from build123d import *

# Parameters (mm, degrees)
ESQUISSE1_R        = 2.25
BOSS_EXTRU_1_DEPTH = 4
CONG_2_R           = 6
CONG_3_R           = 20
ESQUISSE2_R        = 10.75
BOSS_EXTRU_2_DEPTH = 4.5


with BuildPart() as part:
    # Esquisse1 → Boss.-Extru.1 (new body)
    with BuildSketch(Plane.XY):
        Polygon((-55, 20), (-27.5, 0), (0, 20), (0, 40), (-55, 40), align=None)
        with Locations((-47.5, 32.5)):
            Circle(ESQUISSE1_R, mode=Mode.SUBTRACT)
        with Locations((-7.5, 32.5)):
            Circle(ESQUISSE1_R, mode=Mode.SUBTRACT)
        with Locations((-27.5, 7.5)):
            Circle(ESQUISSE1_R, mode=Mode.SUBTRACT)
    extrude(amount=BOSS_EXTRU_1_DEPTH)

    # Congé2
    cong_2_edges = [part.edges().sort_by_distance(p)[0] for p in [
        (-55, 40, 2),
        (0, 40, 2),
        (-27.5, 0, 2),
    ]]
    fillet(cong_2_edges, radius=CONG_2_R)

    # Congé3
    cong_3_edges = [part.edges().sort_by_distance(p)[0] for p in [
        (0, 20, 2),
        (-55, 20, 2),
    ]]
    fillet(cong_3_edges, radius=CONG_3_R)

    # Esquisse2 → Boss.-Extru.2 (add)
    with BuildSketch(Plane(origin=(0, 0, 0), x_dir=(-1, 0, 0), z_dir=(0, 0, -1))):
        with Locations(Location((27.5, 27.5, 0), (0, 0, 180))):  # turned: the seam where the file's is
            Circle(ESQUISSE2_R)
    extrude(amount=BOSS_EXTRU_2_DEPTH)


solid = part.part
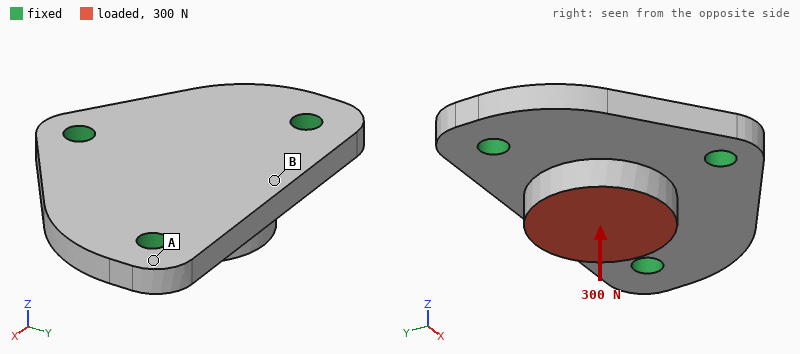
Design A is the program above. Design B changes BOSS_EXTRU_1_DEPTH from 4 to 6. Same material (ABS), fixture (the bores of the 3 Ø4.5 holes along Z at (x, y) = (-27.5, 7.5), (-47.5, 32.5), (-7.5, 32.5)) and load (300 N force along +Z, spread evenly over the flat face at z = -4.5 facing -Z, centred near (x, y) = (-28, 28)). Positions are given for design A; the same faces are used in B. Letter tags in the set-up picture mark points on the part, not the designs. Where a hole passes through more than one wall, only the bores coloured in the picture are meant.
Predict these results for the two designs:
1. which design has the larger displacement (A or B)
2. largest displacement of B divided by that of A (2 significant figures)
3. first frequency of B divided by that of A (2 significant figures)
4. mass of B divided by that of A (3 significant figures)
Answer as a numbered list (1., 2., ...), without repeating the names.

1. A
2. 0.45
3. 1.3
4. 1.40
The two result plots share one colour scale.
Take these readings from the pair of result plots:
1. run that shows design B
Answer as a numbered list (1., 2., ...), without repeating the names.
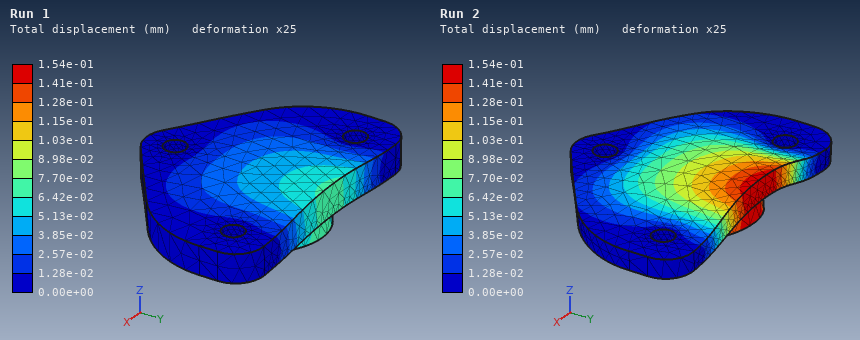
1. Run 1
